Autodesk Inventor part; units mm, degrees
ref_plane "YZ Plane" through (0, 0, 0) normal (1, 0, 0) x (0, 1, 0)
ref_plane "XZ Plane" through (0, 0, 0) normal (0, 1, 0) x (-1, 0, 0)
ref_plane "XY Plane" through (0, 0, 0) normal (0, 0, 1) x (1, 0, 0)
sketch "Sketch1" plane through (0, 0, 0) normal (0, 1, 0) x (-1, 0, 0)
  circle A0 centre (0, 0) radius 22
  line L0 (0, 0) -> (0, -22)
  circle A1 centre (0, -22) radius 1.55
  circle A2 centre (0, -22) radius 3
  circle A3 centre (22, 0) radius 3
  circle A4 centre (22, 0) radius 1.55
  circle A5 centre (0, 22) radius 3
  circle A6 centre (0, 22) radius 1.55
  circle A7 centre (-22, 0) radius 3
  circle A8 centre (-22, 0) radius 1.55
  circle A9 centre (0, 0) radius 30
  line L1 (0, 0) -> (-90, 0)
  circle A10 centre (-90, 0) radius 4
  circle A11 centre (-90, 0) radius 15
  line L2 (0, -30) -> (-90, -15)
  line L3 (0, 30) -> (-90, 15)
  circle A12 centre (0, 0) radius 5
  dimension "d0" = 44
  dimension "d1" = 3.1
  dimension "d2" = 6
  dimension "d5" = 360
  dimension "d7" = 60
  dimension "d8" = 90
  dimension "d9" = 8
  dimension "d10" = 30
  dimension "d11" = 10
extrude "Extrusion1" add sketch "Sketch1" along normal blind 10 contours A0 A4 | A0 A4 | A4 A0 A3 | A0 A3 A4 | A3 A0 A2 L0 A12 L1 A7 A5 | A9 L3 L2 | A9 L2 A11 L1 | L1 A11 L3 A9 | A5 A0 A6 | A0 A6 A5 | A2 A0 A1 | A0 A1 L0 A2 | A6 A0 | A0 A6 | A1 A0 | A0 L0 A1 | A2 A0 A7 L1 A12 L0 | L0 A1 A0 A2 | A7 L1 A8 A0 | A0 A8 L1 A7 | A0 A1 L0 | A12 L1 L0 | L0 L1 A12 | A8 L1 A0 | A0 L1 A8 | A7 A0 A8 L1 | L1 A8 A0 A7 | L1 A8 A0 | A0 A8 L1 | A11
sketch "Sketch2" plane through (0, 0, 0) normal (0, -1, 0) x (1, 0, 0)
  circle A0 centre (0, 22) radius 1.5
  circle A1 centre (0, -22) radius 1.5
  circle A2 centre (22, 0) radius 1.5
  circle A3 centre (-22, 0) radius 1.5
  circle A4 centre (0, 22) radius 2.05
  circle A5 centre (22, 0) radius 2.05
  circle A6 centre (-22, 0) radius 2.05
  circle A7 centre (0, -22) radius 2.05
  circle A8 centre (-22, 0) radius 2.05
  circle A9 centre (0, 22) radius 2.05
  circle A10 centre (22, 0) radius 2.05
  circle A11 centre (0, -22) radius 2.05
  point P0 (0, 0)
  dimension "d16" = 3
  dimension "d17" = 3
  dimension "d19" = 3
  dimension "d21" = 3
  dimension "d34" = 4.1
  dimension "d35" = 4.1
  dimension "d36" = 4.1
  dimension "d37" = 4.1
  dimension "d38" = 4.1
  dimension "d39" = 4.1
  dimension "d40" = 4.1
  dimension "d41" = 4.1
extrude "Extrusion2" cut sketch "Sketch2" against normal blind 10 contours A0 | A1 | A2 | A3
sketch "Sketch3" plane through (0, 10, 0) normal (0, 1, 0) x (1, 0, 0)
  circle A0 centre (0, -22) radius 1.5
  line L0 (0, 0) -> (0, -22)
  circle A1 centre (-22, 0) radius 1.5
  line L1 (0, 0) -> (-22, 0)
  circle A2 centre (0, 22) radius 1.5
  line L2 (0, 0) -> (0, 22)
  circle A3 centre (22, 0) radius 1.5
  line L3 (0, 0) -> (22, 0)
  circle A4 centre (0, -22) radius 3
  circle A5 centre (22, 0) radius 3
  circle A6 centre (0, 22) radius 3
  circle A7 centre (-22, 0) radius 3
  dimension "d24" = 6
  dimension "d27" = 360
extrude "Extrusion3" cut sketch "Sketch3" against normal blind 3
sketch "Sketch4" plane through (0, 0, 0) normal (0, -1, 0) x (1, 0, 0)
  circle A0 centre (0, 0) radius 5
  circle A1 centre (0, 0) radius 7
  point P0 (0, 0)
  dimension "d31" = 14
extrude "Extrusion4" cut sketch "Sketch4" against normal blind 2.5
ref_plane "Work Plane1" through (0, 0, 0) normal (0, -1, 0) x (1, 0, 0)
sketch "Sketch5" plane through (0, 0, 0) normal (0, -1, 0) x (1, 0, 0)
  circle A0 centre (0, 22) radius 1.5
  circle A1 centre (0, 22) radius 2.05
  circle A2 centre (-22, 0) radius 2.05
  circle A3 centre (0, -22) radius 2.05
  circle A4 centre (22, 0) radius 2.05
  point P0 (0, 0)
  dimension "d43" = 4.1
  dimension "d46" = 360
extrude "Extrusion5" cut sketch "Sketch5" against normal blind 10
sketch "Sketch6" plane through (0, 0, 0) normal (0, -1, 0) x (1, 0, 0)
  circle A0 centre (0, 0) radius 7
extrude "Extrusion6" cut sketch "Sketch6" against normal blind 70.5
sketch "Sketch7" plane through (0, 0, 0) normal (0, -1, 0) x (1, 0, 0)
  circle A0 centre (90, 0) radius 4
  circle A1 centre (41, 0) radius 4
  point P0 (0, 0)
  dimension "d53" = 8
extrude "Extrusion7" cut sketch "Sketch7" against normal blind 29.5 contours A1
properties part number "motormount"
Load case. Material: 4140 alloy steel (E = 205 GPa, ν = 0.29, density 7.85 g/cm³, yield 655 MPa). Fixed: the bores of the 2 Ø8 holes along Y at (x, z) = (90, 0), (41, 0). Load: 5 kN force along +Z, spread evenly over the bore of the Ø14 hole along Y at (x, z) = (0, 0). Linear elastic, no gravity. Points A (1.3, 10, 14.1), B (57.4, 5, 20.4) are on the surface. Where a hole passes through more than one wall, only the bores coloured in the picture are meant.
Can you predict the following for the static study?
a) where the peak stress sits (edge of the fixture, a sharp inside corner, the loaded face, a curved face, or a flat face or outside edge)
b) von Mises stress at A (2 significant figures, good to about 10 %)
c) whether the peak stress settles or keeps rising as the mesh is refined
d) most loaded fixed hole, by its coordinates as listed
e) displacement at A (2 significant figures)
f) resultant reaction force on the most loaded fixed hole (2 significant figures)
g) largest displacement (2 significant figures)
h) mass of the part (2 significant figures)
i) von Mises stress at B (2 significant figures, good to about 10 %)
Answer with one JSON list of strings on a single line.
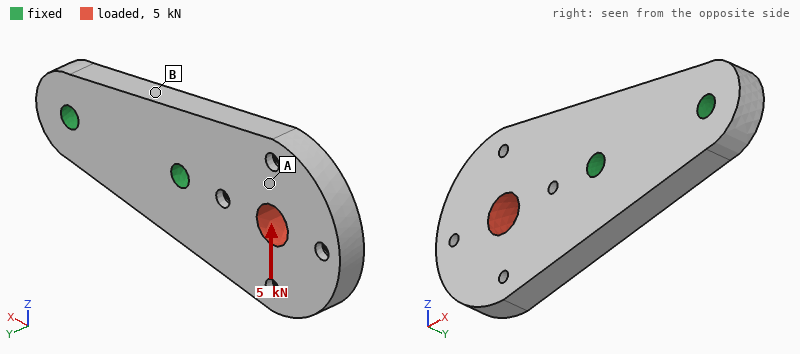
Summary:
["edge of the fixture", "21 MPa", "keeps rising", "(41, 0)", "26 µm", "8.2 kN", "43 µm", "430 g", "42 MPa"]
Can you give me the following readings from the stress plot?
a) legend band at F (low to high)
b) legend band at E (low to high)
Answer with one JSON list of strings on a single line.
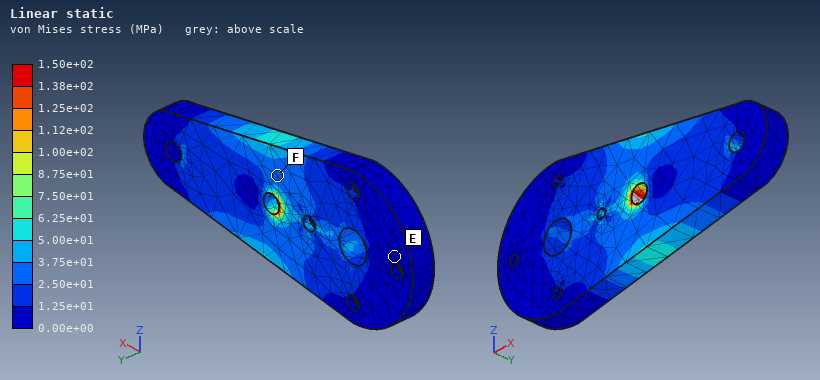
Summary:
["2.50e+01 to 3.75e+01 MPa", "0.00e+00 to 1.25e+01 MPa"]
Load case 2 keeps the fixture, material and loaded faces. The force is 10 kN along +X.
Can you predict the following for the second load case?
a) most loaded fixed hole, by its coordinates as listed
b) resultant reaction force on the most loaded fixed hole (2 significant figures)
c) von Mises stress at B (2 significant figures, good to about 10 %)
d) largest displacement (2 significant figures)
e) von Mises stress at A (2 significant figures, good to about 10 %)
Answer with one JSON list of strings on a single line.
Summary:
["(41, 0)", "8.4 kN", "11 MPa", "7.9 µm", "15 MPa"]
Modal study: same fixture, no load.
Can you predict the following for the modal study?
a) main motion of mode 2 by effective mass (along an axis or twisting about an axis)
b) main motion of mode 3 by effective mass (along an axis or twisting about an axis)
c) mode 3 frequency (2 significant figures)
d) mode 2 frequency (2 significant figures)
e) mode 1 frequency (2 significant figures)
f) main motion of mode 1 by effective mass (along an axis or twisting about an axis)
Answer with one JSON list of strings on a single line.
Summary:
["twisting about X", "along Z", "4300 Hz", "3900 Hz", "1700 Hz", "along Y"]
